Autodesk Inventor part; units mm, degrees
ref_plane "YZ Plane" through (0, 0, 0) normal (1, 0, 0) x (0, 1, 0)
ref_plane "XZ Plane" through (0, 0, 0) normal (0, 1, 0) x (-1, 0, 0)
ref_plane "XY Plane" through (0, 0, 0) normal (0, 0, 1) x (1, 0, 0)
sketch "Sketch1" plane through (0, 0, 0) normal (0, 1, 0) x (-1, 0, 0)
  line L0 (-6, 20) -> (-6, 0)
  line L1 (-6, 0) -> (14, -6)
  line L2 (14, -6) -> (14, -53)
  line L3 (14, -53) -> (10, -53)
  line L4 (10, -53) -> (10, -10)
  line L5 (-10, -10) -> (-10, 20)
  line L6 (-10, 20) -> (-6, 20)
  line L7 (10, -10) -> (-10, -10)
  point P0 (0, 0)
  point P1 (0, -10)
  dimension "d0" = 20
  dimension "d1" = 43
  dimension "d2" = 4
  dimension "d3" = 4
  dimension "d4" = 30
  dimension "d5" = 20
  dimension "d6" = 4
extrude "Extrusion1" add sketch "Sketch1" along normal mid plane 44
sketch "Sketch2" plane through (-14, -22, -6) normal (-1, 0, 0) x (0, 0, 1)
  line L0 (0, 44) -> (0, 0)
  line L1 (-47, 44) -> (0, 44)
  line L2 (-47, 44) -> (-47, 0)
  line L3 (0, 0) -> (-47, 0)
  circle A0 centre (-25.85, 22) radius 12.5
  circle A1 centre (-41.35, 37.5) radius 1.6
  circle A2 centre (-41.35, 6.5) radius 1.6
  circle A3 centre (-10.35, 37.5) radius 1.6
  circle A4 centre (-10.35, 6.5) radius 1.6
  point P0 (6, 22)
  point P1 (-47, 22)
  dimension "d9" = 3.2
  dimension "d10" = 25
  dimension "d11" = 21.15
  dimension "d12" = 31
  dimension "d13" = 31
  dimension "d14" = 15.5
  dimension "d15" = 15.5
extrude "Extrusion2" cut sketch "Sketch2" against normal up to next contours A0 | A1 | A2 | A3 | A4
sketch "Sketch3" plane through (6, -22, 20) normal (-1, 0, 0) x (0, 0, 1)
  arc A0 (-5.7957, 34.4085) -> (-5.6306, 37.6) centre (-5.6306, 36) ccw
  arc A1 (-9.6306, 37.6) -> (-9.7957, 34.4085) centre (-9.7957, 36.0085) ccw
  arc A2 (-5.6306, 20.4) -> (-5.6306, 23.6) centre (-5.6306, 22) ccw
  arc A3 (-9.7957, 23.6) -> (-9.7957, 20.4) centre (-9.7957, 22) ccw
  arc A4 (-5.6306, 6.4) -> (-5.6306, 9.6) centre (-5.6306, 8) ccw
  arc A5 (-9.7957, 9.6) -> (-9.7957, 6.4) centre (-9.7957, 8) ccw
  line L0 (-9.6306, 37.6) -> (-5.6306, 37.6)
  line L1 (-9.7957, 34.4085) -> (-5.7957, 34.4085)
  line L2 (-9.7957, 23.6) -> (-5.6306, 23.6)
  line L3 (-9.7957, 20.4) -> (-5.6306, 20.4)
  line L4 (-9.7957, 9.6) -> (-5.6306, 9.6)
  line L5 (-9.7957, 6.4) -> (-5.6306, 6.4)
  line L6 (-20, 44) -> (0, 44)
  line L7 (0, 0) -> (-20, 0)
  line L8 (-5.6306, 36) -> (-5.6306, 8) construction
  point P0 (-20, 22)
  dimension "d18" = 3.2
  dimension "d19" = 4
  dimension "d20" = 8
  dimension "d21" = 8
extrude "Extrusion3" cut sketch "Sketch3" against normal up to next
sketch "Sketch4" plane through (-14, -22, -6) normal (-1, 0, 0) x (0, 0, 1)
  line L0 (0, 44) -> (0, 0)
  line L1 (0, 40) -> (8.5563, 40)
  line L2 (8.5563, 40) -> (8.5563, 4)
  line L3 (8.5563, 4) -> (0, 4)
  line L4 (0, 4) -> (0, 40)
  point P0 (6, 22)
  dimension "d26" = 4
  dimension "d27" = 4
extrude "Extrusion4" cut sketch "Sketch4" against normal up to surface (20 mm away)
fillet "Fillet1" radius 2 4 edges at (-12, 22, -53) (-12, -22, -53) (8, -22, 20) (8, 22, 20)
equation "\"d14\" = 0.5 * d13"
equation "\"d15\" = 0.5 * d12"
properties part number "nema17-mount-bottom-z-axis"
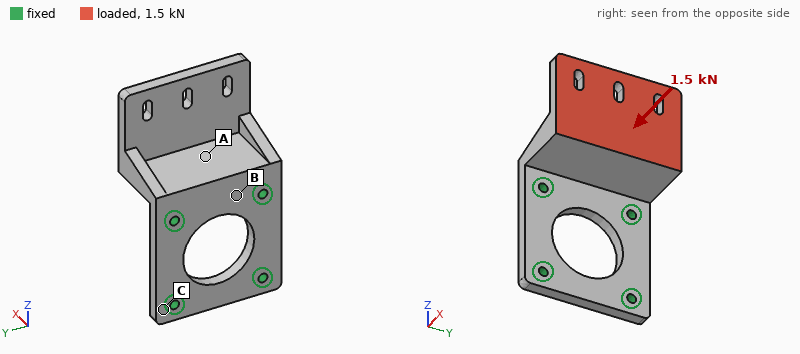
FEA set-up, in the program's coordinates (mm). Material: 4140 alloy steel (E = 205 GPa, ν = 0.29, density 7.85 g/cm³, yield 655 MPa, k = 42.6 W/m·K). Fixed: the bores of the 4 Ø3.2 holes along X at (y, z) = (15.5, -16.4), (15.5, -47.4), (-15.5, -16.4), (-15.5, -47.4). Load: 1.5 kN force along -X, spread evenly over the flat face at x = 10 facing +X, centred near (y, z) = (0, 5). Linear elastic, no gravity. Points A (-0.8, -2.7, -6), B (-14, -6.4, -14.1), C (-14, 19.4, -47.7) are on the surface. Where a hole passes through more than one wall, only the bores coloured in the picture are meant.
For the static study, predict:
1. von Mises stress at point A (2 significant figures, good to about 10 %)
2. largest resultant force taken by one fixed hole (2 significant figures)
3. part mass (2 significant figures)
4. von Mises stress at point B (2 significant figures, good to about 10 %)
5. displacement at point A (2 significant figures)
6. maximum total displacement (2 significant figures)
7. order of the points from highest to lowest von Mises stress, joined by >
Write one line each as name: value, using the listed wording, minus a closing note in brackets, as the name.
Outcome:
von Mises stress at point A: 87 MPa
largest resultant force taken by one fixed hole: 840 N
part mass: 110 g
von Mises stress at point B: 120 MPa
displacement at point A: 0.083 mm
maximum total displacement: 0.37 mm
order of the points from highest to lowest von Mises stress, joined by >: B > A > C
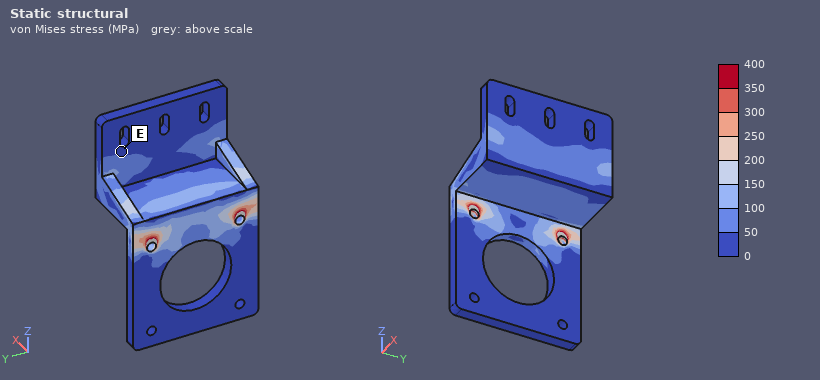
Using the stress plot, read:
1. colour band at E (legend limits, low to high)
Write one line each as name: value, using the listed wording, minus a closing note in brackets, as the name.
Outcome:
colour band at E: 0 to 50 MPa
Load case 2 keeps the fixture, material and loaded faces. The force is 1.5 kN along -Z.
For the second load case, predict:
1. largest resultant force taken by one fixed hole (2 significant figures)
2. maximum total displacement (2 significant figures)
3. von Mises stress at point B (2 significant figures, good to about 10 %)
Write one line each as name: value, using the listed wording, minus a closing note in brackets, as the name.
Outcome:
largest resultant force taken by one fixed hole: 790 N
maximum total displacement: 0.39 mm
von Mises stress at point B: 160 MPa
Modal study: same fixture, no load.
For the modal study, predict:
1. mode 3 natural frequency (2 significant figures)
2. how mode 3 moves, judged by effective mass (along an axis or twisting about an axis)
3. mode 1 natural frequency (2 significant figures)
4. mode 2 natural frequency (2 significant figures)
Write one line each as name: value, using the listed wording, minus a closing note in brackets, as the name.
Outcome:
mode 3 natural frequency: 6000 Hz
how mode 3 moves, judged by effective mass: along Z
mode 1 natural frequency: 1600 Hz
mode 2 natural frequency: 3700 Hz
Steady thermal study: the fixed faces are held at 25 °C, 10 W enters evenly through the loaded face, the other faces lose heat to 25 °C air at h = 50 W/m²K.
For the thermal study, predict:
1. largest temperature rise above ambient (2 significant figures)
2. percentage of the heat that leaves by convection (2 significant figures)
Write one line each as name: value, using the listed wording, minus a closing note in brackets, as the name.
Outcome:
largest temperature rise above ambient: 33 K
percentage of the heat that leaves by convection: 44 %
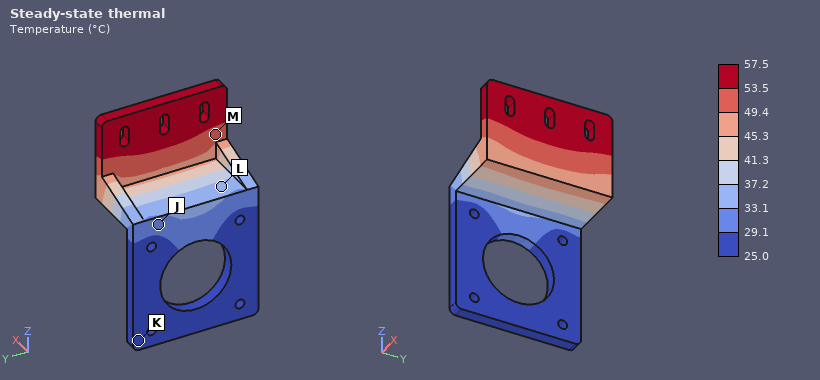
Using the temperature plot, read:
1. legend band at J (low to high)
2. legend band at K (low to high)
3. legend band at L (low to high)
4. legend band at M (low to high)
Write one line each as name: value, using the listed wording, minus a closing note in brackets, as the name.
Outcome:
legend band at J: 29.1 to 33.1 °C
legend band at K: 25.0 to 29.1 °C
legend band at L: 33.1 to 37.2 °C
legend band at M: 49.4 to 53.5 °C
